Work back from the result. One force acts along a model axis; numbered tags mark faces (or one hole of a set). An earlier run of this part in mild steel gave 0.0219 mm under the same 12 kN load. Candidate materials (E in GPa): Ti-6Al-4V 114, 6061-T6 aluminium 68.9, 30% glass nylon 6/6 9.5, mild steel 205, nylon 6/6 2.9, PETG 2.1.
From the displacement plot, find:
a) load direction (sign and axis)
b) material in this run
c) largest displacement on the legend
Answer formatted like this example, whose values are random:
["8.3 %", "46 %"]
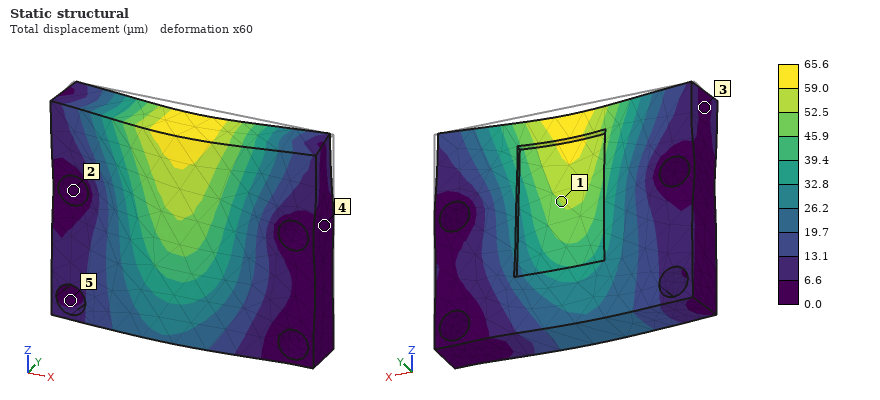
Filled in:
["-Y", "6061-T6 aluminium", "65.6 µm"]
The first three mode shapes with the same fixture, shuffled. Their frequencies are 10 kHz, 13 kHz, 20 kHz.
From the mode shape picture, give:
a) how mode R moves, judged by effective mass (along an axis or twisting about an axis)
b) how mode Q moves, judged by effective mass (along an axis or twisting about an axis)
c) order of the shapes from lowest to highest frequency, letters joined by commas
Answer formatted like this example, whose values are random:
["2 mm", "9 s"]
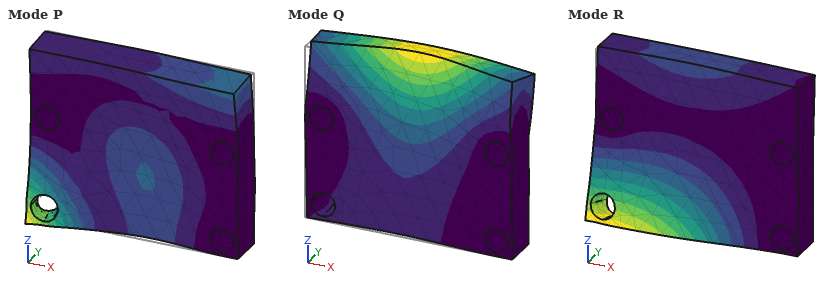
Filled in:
["along Y", "along Y", "R, Q, P"]
